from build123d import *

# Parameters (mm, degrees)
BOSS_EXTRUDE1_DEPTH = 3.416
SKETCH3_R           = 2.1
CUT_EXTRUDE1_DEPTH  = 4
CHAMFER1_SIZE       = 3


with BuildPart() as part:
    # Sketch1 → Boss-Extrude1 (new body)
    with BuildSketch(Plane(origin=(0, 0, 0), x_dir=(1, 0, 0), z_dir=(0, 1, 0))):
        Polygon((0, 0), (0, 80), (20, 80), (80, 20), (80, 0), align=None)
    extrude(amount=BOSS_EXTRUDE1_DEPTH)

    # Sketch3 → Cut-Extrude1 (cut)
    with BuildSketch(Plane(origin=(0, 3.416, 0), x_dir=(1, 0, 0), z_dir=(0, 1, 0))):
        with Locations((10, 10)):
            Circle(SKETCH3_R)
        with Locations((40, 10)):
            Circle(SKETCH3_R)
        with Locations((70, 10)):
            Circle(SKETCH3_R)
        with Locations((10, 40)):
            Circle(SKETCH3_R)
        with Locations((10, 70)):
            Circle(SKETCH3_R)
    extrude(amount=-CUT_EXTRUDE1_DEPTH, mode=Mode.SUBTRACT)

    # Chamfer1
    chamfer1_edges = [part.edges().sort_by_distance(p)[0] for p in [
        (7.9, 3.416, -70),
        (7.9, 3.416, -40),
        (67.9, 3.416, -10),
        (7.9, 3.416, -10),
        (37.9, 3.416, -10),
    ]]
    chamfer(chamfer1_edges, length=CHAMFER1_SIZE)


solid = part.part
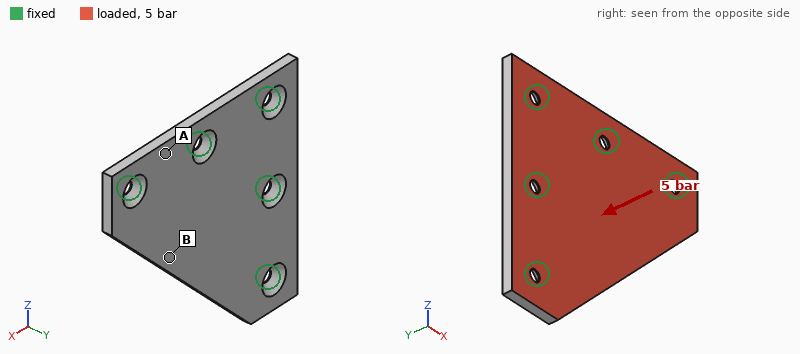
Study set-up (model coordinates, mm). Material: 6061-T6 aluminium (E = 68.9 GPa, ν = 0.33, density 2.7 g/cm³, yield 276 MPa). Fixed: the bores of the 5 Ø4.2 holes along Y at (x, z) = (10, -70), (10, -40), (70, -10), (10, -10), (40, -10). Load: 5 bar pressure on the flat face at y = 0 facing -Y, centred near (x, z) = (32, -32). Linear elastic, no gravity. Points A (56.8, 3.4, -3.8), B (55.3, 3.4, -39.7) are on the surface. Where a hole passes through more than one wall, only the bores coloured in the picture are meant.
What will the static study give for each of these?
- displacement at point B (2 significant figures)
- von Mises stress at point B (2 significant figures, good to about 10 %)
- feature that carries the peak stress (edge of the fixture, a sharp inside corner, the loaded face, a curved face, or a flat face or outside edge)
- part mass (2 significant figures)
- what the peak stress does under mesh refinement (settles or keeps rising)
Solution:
0.34 mm
63 MPa
edge of the fixture
41 g
keeps rising
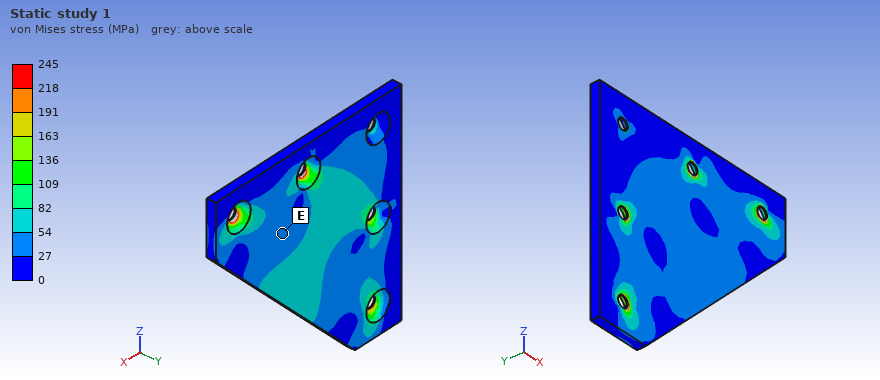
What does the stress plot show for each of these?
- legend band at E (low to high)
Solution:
27 to 54 MPa
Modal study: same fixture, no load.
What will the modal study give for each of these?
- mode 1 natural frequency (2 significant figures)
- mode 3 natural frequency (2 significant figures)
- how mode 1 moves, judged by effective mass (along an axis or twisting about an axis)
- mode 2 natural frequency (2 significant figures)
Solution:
2400 Hz
8400 Hz
along Y
5100 Hz
